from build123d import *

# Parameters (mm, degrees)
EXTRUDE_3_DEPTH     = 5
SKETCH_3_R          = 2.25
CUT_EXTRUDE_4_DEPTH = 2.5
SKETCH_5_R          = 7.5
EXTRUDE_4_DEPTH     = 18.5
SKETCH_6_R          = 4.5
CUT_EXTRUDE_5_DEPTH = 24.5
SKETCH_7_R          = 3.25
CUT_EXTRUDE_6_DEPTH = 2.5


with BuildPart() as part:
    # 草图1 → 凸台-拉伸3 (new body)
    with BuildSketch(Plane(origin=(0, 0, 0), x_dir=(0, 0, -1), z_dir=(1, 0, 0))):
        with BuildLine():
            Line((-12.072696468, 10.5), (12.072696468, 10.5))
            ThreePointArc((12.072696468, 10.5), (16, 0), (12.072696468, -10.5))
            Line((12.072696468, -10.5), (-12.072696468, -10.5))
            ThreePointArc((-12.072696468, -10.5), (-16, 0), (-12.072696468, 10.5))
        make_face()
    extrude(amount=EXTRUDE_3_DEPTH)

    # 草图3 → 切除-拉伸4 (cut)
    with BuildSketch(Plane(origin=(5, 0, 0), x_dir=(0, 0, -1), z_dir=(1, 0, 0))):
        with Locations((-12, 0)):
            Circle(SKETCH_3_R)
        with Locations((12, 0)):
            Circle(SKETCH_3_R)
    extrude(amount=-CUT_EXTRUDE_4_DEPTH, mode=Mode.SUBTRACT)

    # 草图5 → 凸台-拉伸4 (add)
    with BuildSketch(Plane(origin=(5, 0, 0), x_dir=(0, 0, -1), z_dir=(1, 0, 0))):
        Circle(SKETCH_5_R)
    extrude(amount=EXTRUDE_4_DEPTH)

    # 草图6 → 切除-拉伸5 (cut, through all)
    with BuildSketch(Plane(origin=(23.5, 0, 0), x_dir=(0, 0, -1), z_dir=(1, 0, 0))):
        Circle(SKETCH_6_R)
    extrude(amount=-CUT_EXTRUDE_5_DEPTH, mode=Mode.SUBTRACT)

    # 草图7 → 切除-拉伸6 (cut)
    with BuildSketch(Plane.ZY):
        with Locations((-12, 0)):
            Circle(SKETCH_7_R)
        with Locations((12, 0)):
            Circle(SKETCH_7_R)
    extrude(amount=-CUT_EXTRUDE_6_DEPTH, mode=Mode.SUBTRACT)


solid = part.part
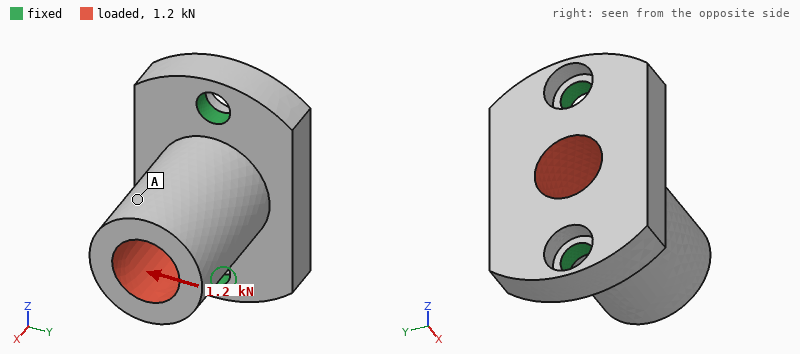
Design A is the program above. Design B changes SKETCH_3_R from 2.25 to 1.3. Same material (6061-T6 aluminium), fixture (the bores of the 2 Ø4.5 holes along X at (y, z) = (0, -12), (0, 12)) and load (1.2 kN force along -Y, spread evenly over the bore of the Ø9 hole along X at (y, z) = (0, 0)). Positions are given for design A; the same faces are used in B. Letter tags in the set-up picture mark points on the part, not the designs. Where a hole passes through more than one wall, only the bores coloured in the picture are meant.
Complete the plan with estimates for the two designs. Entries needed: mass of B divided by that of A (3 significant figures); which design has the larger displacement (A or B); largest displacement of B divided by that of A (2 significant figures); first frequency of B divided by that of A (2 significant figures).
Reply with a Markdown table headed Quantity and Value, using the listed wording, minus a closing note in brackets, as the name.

| Quantity | Value |
|---|---|
| mass of B divided by that of A | 1.01 |
| which design has the larger displacement | B |
| largest displacement of B divided by that of A | 1.7 |
| first frequency of B divided by that of A | 0.75 |
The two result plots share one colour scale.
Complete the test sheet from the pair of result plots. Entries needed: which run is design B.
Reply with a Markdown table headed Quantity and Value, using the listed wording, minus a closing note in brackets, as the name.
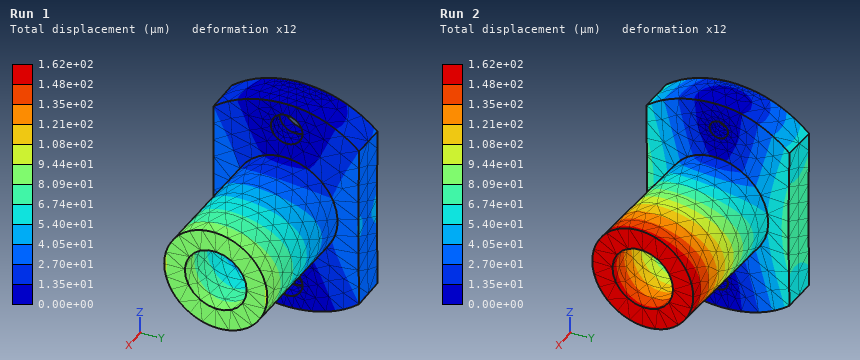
| Quantity | Value |
|---|---|
| which run is design B | Run 2 |
